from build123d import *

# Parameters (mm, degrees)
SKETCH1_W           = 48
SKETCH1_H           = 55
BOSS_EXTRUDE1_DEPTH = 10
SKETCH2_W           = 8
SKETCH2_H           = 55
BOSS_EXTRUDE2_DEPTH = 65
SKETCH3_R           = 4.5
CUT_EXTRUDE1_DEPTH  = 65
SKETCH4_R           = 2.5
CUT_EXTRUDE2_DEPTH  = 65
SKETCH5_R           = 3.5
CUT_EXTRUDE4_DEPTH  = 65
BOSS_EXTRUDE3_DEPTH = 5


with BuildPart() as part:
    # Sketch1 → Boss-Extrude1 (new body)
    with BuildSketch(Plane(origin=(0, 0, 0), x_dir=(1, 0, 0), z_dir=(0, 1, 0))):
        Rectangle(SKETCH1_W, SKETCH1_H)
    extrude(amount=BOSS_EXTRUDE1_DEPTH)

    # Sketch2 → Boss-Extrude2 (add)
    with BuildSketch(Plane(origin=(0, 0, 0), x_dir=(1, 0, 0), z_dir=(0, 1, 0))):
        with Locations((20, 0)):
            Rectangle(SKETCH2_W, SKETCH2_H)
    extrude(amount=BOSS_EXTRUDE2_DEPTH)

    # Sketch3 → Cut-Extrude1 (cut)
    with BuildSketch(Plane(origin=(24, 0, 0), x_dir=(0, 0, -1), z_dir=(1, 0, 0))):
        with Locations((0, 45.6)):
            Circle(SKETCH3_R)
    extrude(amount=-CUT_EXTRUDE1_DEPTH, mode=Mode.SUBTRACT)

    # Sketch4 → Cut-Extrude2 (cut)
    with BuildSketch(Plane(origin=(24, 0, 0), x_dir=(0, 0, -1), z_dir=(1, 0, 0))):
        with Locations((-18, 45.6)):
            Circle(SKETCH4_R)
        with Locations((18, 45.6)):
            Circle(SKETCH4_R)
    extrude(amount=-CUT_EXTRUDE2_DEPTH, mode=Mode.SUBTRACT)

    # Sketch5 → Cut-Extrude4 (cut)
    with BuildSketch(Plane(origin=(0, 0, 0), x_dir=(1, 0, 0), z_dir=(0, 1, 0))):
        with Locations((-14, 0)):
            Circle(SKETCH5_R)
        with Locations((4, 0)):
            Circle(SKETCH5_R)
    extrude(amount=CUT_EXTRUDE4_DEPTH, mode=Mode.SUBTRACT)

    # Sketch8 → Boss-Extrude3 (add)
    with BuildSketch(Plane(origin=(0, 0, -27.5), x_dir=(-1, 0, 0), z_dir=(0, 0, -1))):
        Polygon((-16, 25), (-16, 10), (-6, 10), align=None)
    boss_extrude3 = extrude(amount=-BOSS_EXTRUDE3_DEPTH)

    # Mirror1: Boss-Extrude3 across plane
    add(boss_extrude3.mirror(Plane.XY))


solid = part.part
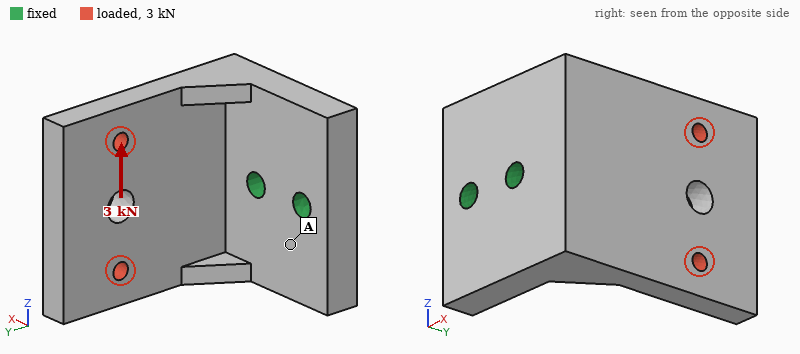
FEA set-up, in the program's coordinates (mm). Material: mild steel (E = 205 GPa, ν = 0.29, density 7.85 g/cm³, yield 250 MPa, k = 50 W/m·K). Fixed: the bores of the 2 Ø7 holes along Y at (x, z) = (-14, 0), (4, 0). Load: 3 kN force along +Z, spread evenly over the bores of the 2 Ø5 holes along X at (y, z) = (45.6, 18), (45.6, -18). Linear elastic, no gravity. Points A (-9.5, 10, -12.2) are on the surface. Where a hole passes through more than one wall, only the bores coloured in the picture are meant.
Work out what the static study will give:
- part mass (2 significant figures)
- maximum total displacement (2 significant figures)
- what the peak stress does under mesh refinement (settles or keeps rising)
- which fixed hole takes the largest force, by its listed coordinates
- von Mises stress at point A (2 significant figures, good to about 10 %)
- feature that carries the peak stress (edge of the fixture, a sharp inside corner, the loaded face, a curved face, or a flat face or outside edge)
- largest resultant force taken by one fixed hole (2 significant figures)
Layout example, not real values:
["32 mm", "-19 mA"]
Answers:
["390 g", "0.11 mm", "keeps rising", "(4, 0)", "41 MPa", "edge of the fixture", "4.7 kN"]
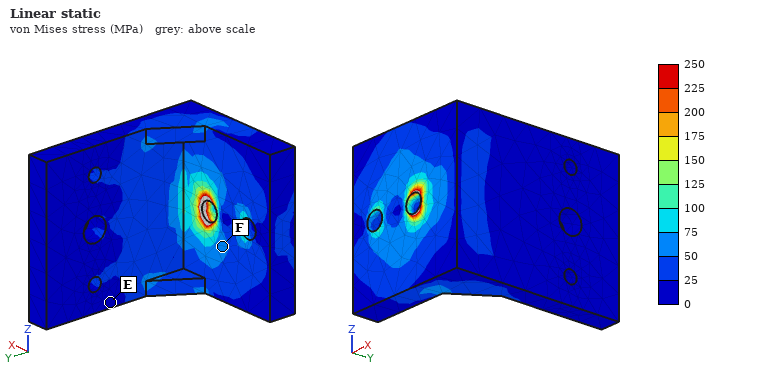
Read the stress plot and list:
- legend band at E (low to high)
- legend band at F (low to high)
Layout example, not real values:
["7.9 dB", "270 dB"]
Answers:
["0 to 25 MPa", "50 to 75 MPa"]
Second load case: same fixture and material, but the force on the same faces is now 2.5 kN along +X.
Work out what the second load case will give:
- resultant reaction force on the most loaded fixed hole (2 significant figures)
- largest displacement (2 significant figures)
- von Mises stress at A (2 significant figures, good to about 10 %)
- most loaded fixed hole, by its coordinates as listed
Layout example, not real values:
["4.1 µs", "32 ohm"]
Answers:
["3.1 kN", "0.22 mm", "25 MPa", "(4, 0)"]
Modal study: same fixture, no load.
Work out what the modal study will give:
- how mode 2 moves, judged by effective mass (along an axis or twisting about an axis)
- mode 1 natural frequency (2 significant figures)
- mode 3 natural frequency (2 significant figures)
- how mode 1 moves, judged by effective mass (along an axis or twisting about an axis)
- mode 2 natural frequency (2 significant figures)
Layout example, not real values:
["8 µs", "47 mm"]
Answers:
["along Z", "1700 Hz", "4700 Hz", "along X", "2500 Hz"]
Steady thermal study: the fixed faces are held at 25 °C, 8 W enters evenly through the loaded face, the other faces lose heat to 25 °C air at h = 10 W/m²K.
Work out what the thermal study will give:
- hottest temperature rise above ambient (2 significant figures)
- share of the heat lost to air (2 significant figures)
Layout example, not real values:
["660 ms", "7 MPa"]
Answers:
["19 K", "15 %"]
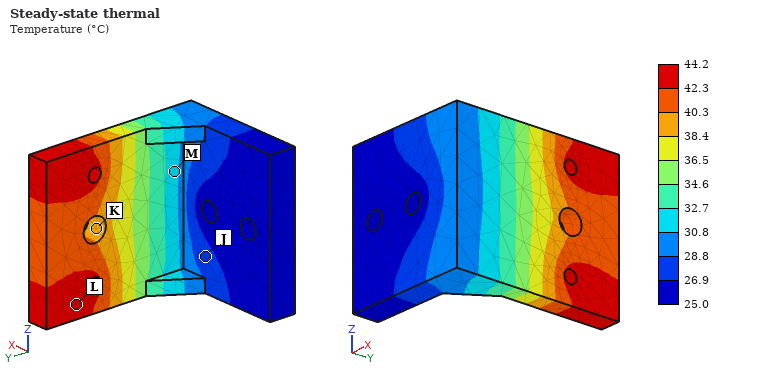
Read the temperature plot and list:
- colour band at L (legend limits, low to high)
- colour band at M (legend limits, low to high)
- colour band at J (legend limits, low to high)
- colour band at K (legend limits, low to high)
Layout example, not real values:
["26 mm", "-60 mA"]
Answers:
["42.3 to 44.2 °C", "30.8 to 32.7 °C", "26.9 to 28.8 °C", "38.4 to 40.3 °C"]
